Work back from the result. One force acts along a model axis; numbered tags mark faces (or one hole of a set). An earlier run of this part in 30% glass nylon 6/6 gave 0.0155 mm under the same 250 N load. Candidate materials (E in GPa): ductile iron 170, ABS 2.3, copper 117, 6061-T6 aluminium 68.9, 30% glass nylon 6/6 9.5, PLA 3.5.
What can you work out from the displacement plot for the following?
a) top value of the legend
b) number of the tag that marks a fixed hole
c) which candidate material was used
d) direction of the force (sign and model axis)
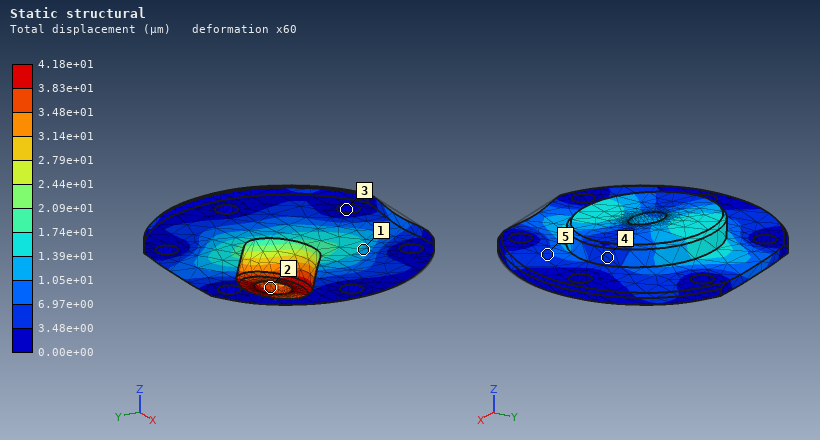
4.18e+01 µm
3
PLA
+Y
